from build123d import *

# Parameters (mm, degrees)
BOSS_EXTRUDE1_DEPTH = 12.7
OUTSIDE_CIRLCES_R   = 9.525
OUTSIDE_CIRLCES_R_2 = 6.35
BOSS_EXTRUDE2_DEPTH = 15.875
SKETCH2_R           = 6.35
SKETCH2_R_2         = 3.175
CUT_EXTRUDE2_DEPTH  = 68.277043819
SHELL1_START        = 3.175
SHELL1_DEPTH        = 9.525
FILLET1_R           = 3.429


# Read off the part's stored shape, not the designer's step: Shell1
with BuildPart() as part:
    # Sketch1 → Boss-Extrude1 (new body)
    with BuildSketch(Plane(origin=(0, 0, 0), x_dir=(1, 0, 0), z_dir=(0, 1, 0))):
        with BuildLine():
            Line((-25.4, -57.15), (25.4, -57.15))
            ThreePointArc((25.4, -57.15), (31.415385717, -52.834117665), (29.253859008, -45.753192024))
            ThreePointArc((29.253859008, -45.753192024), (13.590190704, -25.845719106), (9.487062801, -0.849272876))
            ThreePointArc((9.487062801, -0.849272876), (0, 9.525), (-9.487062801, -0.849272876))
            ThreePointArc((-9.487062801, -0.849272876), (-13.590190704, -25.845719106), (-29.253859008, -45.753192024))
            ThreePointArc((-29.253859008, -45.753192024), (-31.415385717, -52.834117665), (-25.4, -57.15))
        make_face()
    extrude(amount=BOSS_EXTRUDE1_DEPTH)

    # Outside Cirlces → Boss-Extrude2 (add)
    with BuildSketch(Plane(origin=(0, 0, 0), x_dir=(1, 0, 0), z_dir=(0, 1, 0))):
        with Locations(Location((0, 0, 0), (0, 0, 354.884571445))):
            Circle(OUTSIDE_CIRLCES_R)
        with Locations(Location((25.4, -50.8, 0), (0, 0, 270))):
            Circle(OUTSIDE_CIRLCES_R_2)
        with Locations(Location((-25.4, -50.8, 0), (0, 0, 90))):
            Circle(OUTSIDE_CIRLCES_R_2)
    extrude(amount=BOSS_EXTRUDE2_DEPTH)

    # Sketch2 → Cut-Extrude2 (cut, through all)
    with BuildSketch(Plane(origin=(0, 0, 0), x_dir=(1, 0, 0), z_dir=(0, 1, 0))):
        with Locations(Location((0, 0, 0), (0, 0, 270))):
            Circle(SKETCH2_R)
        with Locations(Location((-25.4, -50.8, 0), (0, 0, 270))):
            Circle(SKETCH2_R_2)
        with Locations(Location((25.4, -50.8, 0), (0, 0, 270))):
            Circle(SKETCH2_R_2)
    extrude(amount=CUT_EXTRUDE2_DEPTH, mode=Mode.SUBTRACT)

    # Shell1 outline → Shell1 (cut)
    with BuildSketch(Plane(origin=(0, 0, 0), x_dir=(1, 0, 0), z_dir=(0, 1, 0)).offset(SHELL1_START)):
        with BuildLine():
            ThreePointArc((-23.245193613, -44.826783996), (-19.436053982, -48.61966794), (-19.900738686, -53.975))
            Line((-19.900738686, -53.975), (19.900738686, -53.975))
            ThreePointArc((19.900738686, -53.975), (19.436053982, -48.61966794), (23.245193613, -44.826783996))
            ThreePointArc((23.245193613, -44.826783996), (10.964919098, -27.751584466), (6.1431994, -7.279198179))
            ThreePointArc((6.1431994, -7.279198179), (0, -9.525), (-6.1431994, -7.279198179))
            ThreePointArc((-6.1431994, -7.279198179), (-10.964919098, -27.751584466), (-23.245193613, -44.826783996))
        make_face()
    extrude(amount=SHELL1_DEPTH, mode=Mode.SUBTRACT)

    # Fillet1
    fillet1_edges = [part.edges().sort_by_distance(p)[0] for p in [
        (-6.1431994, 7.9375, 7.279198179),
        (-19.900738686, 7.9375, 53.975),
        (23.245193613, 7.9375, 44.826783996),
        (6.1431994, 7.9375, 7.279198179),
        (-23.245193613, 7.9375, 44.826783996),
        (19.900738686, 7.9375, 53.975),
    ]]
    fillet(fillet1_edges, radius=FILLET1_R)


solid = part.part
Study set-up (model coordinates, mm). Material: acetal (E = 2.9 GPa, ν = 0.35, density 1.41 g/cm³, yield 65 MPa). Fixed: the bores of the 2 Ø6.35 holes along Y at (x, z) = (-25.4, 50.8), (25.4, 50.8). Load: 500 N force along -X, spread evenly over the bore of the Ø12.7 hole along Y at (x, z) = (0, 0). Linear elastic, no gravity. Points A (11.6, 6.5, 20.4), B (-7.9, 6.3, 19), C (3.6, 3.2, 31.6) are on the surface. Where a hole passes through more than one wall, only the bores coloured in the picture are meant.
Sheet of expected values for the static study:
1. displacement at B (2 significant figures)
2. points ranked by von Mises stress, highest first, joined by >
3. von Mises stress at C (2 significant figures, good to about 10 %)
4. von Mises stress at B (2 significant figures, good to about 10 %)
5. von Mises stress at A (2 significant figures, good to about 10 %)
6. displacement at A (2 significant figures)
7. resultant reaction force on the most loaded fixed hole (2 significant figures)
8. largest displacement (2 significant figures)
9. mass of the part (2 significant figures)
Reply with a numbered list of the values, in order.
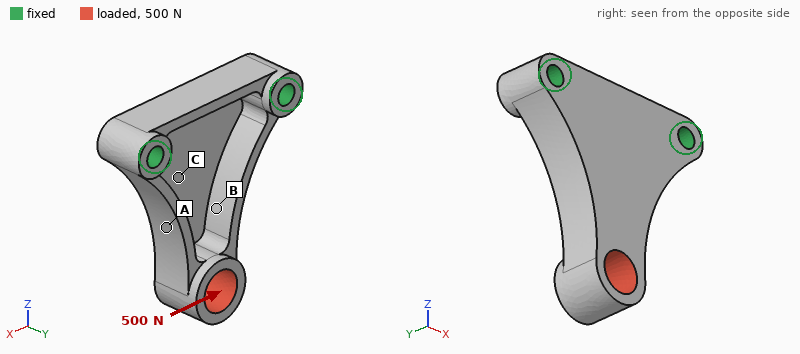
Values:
1. 0.23 mm
2. A > B > C
3. 4.5 MPa
4. 11 MPa
5. 22 MPa
6. 0.22 mm
7. 560 N
8. 1.0 mm
9. 21 g
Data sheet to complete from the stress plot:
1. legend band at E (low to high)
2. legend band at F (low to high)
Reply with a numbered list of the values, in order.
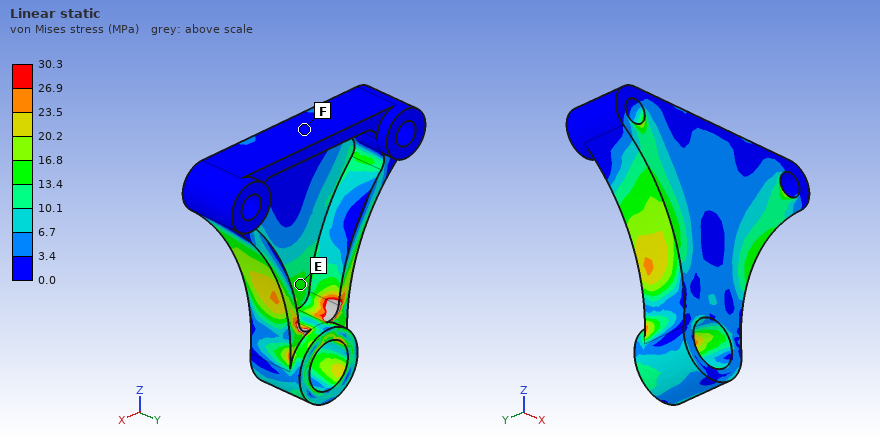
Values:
1. 13.4 to 16.8 MPa
2. 0.0 to 3.4 MPa
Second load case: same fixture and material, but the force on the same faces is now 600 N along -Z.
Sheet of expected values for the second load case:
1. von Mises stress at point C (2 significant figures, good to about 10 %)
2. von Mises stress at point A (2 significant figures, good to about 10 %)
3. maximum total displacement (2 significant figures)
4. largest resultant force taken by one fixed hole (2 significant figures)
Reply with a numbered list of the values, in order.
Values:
1. 6.4 MPa
2. 11 MPa
3. 1.00 mm
4. 340 N
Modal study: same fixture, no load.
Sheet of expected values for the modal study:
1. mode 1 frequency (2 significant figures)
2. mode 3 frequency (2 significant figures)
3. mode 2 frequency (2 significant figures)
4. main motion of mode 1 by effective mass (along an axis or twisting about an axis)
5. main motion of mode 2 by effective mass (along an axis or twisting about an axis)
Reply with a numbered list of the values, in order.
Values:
1. 710 Hz
2. 2500 Hz
3. 1800 Hz
4. along Y
5. along X
